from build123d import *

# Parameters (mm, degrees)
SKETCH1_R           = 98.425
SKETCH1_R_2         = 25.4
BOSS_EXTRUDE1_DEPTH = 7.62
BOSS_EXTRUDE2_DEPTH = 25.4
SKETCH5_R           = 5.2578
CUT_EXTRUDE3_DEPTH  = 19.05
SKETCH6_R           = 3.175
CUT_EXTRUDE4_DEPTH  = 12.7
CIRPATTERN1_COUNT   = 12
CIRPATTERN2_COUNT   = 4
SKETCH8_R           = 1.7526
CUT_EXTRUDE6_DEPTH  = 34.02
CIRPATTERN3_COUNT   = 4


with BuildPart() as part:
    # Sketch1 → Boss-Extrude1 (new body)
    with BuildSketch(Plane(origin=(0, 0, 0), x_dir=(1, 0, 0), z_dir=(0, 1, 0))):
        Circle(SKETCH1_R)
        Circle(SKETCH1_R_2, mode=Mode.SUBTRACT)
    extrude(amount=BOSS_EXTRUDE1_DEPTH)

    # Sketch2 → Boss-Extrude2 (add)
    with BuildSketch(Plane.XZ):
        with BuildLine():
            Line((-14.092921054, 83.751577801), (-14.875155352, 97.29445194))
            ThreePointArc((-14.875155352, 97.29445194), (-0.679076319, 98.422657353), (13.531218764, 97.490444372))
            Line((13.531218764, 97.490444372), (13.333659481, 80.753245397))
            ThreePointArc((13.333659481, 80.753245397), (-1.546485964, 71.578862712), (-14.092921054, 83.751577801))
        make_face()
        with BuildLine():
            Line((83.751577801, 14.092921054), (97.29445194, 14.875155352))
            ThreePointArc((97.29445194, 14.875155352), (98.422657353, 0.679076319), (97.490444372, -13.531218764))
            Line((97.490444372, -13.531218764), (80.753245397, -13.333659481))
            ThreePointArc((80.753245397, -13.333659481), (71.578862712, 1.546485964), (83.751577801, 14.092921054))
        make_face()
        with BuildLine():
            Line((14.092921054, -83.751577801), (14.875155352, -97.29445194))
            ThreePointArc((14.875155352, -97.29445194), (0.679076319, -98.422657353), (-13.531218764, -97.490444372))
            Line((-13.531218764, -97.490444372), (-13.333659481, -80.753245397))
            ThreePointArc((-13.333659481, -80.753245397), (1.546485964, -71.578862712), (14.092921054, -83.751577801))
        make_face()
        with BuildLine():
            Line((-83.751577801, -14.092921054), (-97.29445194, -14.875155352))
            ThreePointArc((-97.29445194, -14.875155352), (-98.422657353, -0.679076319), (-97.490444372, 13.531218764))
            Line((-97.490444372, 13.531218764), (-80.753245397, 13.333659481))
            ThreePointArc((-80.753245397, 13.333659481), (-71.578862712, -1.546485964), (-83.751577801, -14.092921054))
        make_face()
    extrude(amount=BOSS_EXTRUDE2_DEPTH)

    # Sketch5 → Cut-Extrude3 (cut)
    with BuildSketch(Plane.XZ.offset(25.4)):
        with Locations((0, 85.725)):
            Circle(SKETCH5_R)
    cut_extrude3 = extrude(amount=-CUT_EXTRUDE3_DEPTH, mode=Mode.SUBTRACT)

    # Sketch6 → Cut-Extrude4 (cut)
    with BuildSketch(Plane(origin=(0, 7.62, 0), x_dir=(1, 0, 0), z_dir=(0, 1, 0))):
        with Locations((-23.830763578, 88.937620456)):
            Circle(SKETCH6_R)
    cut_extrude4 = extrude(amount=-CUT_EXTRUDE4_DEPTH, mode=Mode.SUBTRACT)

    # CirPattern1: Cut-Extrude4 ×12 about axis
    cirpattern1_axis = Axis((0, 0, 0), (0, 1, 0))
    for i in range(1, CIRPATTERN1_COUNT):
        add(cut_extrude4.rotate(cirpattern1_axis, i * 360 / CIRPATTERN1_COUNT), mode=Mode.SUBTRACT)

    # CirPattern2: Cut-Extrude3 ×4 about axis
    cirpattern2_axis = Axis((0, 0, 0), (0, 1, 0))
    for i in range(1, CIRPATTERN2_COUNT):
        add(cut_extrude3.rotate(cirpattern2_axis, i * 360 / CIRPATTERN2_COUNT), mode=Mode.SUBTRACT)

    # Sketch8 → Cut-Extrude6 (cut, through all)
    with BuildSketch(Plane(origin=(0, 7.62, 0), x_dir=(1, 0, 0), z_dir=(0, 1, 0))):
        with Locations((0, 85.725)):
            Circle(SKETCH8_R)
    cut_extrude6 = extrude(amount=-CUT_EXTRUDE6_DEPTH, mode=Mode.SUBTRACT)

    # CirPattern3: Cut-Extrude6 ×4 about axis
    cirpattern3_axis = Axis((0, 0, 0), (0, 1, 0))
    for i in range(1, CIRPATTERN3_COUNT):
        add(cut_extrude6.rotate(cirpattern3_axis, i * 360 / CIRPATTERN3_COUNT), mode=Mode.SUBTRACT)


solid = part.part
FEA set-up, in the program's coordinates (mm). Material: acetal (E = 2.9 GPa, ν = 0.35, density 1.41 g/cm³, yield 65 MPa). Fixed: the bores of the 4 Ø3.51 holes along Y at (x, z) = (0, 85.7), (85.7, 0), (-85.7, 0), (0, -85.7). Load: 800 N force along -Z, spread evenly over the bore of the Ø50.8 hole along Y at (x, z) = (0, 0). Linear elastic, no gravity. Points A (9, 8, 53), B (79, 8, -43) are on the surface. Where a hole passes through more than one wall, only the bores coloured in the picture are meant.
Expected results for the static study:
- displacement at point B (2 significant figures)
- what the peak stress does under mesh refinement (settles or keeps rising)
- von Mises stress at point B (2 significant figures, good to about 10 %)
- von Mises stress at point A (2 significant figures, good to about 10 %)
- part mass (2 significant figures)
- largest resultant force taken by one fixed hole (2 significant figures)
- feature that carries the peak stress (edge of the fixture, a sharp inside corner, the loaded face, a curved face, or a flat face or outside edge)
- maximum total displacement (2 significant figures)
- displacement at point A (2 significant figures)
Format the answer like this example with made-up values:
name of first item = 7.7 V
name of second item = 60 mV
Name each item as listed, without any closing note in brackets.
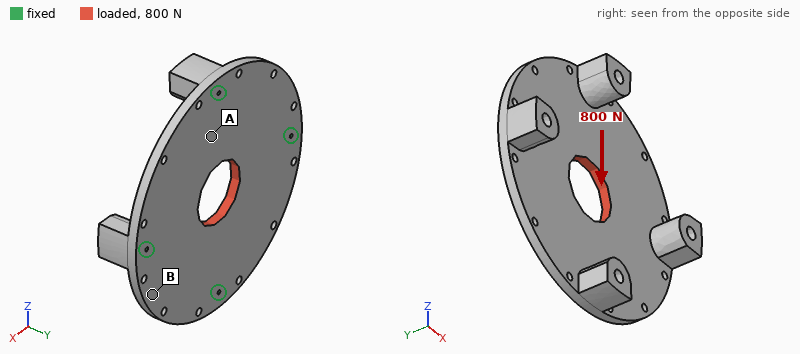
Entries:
displacement at point B = 10 µm
what the peak stress does under mesh refinement = keeps rising
von Mises stress at point B = 0.23 MPa
von Mises stress at point A = 0.81 MPa
part mass = 390 g
largest resultant force taken by one fixed hole = 250 N
feature that carries the peak stress = edge of the fixture
maximum total displacement = 23 µm
displacement at point A = 14 µm
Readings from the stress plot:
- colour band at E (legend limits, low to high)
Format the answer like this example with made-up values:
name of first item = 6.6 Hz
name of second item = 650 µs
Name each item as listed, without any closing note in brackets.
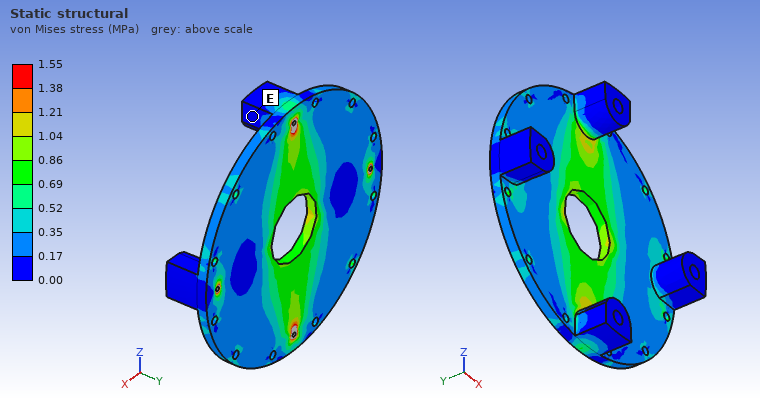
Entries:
colour band at E = 0.00 to 0.17 MPa
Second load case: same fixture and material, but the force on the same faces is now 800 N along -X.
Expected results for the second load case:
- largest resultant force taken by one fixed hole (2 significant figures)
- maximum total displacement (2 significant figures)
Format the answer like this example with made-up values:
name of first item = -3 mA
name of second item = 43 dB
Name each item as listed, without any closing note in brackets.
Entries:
largest resultant force taken by one fixed hole = 250 N
maximum total displacement = 23 µm
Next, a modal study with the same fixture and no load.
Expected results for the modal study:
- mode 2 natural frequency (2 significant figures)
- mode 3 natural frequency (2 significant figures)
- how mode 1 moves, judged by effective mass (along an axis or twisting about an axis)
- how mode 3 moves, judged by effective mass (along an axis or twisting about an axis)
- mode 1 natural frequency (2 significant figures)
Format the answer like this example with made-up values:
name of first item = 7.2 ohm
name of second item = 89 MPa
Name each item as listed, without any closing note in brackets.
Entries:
mode 2 natural frequency = 690 Hz
mode 3 natural frequency = 740 Hz
how mode 1 moves, judged by effective mass = along Y
how mode 3 moves, judged by effective mass = twisting about X
mode 1 natural frequency = 660 Hz
